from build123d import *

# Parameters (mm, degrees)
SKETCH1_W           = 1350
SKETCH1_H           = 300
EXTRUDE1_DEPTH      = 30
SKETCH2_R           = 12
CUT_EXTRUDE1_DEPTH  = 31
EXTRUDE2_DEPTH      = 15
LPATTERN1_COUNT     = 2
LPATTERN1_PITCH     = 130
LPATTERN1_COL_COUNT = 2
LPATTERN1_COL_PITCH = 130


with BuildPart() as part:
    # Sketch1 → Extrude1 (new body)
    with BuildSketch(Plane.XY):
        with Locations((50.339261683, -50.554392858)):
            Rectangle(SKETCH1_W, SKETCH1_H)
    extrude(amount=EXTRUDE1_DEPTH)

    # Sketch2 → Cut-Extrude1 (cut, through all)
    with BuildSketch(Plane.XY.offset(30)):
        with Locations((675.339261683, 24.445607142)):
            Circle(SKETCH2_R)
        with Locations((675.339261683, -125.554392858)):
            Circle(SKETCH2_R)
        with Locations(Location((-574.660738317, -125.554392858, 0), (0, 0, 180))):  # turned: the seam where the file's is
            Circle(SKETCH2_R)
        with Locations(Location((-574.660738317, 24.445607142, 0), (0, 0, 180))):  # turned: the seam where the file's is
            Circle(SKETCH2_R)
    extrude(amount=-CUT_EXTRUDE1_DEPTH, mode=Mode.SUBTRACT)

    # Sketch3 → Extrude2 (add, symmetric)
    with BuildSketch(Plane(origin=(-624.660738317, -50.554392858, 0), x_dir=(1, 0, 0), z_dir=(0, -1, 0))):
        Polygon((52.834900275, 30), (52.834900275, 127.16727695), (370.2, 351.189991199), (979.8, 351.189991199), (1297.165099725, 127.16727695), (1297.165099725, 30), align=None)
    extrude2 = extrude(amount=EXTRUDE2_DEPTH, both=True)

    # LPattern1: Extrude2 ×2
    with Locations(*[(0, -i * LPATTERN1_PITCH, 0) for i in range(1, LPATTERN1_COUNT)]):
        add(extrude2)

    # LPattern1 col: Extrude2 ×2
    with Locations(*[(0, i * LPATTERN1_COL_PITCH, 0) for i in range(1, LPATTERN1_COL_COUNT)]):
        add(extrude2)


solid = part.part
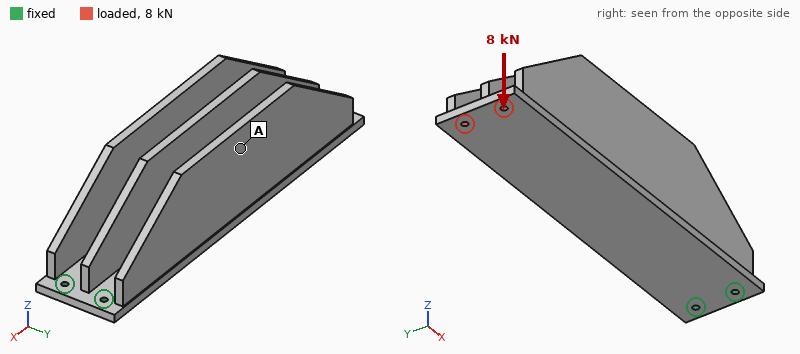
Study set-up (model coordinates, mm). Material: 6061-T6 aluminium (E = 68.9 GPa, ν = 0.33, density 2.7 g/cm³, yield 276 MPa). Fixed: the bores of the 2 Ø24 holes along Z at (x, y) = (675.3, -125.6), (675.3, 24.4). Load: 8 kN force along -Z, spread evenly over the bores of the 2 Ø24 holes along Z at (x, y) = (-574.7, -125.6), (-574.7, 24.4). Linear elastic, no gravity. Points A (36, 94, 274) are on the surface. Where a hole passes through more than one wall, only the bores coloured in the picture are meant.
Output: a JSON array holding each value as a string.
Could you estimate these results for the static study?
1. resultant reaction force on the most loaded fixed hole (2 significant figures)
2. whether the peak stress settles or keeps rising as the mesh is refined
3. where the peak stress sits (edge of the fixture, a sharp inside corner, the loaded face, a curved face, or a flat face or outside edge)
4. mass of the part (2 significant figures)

["6.2 kN", "keeps rising", "edge of the fixture", "110 kg"]
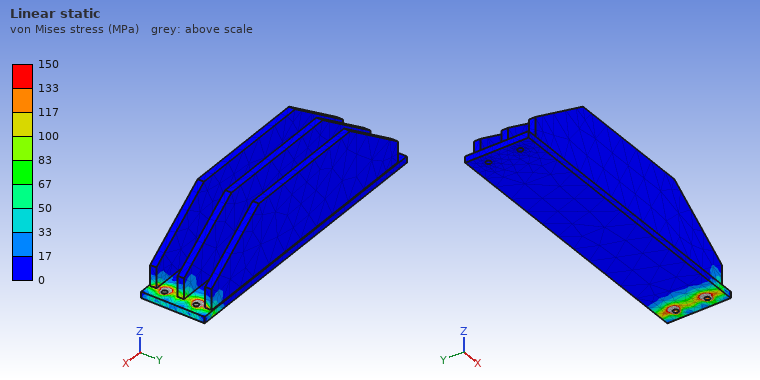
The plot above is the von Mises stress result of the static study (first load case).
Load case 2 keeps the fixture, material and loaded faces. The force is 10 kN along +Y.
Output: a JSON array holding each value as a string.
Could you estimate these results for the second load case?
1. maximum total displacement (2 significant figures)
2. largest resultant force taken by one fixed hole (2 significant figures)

["1.2 mm", "76 kN"]
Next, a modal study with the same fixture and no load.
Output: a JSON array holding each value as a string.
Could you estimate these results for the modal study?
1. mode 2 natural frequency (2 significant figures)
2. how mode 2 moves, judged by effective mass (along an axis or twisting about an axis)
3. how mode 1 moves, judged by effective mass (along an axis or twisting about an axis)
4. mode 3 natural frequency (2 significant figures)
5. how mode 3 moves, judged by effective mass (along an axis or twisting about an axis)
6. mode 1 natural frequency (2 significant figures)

["56 Hz", "along Y", "along Z", "110 Hz", "along Y", "22 Hz"]
